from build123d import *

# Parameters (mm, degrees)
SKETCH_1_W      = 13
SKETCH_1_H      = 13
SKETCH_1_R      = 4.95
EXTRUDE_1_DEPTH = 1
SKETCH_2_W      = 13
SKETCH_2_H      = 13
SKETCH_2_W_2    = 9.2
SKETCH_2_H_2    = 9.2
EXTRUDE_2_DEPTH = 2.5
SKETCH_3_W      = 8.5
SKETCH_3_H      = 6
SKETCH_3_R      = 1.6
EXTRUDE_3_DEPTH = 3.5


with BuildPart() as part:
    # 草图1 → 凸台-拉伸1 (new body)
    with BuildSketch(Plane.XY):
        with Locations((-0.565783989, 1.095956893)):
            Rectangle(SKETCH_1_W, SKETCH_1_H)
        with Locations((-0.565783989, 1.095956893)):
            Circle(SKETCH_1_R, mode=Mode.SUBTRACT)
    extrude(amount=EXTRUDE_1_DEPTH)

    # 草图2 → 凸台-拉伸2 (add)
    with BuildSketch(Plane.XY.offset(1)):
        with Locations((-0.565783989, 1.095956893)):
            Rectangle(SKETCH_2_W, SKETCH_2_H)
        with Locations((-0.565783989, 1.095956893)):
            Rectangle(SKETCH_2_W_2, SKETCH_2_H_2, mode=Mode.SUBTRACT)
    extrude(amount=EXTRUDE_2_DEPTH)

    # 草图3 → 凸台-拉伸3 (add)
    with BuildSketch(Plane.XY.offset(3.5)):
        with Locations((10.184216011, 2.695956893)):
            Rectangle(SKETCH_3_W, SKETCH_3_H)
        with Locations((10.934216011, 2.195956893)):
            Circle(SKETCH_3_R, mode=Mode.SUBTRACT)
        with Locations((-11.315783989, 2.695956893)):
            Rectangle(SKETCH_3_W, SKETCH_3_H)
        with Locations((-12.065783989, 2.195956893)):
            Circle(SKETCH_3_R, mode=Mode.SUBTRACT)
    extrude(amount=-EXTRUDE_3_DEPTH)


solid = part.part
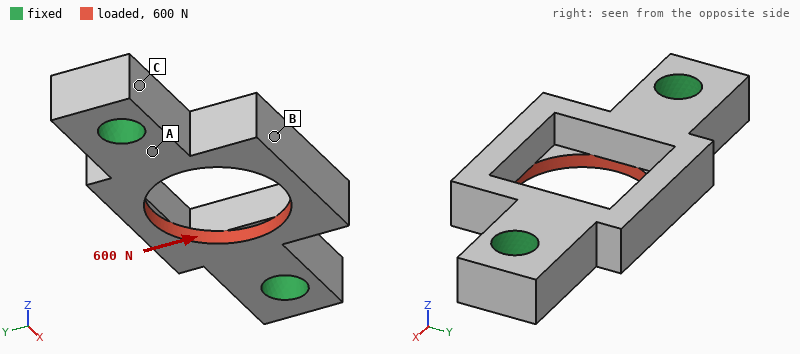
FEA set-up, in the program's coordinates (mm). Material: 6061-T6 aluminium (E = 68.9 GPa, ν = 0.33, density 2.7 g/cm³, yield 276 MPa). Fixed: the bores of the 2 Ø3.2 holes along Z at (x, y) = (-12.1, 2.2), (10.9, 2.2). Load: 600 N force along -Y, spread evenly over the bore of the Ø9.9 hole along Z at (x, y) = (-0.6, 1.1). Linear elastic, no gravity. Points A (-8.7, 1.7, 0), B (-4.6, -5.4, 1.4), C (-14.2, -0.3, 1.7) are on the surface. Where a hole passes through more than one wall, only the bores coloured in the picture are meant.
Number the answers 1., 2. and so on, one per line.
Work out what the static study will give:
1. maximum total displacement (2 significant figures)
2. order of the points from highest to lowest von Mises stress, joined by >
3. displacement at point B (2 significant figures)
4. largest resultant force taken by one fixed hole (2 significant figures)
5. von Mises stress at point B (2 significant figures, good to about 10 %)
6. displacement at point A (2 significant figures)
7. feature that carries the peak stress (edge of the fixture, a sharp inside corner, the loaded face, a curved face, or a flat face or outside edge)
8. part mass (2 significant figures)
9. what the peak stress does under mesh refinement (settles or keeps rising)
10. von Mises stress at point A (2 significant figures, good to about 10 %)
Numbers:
1. 22 µm
2. A > B > C
3. 17 µm
4. 310 N
5. 17 MPa
6. 3.3 µm
7. edge of the fixture
8. 1.6 g
9. keeps rising
10. 68 MPa
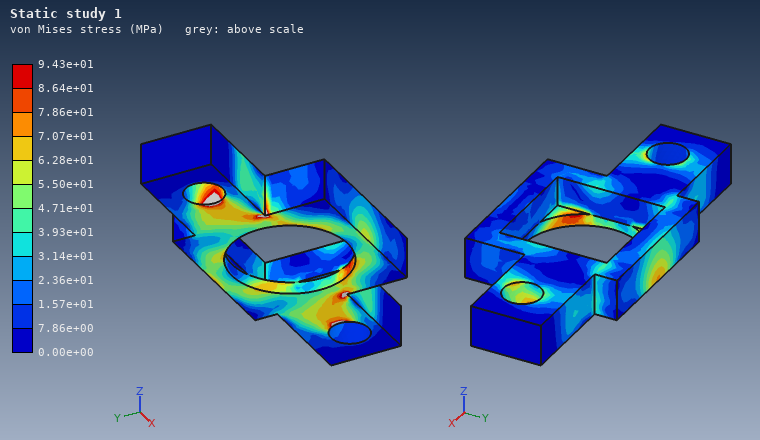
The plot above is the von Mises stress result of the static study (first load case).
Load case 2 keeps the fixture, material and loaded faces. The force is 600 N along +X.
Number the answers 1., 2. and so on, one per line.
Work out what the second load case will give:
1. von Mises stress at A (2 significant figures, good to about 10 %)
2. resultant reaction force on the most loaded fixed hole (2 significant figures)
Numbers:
1. 27 MPa
2. 300 N
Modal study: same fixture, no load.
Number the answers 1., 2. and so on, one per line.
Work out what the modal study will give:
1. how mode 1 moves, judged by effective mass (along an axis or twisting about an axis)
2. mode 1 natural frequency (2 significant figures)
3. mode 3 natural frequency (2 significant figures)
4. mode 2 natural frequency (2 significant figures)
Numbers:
1. along Z
2. 21 kHz
3. 36 kHz
4. 35 kHz
